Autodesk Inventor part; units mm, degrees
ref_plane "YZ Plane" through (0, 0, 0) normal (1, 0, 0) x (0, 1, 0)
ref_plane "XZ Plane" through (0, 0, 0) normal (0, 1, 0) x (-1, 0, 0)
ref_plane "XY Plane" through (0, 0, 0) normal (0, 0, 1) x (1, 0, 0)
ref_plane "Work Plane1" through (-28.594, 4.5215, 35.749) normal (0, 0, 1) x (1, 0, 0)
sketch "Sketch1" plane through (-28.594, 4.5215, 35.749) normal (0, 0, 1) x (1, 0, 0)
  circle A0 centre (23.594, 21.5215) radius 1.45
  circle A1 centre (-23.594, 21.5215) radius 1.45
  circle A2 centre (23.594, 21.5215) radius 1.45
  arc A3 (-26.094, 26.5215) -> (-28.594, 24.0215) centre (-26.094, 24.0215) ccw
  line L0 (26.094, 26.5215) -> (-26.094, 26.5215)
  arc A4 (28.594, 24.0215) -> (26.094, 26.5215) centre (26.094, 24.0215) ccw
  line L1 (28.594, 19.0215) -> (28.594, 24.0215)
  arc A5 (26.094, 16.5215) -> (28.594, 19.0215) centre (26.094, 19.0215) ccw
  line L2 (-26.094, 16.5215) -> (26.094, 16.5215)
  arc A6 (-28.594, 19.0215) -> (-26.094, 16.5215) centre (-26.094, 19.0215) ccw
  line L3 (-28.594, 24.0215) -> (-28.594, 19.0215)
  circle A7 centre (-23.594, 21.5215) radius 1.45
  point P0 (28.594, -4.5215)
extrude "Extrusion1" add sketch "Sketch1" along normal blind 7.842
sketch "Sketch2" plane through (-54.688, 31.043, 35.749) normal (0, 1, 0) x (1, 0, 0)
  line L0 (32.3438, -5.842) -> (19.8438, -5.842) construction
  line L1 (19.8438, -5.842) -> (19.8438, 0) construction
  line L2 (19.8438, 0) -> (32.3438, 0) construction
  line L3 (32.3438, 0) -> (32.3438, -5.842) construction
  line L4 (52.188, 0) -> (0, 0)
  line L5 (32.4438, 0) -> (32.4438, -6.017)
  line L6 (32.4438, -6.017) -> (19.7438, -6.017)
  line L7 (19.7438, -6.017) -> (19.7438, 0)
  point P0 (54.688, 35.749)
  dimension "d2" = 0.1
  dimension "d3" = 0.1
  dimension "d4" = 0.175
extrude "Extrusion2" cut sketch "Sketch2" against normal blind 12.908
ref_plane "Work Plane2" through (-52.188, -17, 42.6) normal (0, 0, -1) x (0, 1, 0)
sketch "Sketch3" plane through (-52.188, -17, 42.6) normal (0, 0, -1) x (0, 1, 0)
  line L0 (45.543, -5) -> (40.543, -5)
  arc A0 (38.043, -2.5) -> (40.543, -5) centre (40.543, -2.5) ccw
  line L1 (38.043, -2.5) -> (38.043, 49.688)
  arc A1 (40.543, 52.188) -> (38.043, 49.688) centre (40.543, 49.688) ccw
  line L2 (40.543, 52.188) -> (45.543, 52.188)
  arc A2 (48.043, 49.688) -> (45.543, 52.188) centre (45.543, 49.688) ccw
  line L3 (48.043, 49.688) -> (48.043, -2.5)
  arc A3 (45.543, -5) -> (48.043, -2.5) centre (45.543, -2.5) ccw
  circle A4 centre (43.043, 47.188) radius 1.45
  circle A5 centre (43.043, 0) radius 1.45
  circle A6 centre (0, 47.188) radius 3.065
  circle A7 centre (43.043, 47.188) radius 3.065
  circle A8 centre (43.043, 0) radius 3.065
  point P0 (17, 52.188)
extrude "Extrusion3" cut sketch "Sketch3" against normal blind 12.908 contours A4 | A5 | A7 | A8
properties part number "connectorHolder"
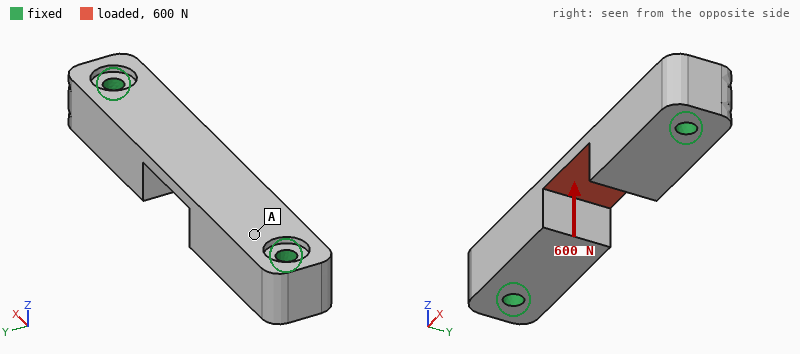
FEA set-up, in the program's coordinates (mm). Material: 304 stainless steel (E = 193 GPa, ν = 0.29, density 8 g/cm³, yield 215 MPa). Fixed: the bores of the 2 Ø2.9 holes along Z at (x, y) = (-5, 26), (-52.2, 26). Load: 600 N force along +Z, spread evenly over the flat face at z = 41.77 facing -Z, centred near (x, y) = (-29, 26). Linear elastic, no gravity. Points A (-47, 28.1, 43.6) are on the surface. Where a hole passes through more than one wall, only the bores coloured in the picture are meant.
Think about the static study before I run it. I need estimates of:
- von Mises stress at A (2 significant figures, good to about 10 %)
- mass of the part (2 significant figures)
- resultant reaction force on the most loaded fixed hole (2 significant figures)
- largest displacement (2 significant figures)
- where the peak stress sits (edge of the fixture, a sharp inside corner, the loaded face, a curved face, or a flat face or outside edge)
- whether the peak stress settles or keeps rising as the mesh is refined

17 MPa
28 g
570 N
14 µm
edge of the fixture
keeps rising
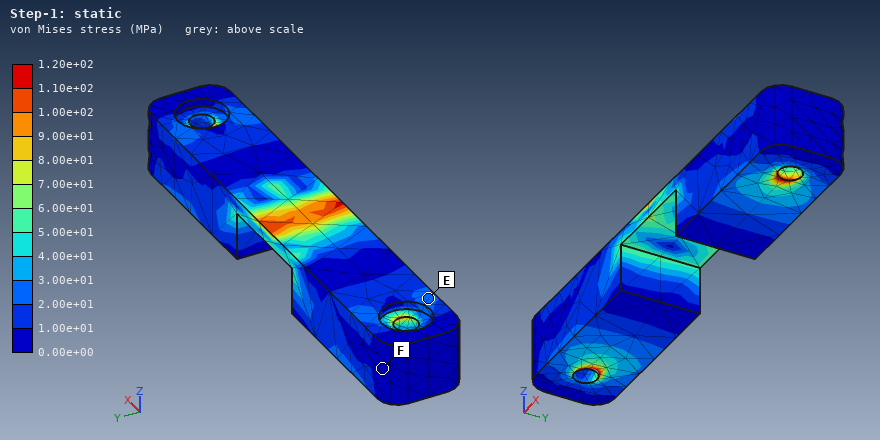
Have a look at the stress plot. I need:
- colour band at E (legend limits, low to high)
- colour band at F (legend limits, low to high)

2.00e+01 to 3.00e+01 MPa
0.00e+00 to 1.00e+01 MPa
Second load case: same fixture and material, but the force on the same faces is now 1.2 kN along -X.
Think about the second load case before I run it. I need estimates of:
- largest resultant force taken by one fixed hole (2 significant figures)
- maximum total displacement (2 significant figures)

600 N
4.7 µm
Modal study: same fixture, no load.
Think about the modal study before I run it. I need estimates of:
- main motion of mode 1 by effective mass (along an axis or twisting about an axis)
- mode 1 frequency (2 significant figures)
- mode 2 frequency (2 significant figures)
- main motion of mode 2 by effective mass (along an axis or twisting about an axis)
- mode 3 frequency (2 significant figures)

along Y
15 kHz
16 kHz
along Z
19 kHz
